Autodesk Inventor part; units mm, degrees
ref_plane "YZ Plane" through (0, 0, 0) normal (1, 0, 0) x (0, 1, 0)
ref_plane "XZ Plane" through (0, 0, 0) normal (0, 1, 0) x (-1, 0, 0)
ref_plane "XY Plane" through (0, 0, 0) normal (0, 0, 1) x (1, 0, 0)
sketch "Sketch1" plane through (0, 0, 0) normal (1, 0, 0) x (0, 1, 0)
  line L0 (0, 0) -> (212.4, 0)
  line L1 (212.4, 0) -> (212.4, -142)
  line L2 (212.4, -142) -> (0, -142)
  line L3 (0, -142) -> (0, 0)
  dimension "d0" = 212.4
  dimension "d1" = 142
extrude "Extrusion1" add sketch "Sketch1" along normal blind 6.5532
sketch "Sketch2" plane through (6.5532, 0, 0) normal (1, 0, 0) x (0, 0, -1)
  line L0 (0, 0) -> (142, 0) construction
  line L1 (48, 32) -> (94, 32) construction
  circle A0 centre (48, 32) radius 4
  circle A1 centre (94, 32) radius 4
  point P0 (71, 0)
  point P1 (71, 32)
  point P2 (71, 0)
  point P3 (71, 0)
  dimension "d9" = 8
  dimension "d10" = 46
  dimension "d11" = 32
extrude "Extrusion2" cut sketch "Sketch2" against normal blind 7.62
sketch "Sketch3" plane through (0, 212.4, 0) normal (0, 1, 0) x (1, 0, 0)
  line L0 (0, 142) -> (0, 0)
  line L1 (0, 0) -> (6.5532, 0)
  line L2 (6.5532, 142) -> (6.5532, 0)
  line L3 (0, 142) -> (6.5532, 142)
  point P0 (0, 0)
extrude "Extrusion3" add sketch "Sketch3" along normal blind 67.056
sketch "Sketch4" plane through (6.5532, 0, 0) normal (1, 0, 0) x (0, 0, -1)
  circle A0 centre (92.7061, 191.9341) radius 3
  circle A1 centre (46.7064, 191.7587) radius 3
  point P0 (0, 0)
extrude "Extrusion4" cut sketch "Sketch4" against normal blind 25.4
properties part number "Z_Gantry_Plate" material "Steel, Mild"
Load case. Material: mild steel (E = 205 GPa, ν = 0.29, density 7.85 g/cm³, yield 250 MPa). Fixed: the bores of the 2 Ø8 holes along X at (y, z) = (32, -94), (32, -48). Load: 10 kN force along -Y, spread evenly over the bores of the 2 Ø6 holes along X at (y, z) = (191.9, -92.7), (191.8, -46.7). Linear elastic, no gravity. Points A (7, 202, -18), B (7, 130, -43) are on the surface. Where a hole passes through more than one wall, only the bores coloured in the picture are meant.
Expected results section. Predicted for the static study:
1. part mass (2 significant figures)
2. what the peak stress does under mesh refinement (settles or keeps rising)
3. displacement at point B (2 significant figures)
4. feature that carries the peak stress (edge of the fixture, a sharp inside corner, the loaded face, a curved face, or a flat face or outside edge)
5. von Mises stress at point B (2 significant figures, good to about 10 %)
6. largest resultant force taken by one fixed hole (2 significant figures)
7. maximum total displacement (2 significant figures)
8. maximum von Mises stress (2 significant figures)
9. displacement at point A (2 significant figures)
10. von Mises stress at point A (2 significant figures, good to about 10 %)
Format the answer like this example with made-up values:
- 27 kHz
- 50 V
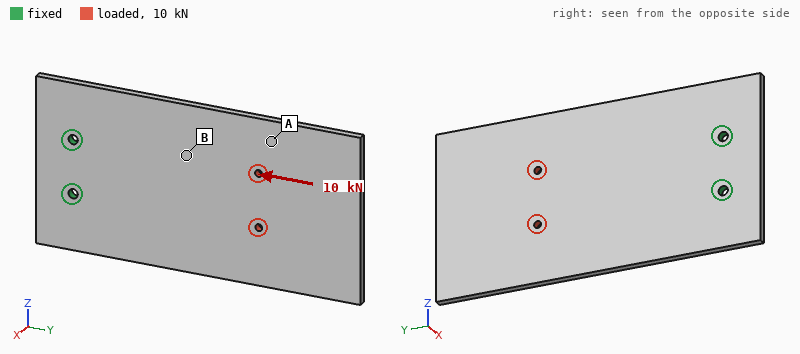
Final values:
- 2.0 kg
- settles
- 7.6 µm
- the loaded face
- 13 MPa
- 5.3 kN
- 13 µm
- 72 MPa
- 10 µm
- 5.2 MPa
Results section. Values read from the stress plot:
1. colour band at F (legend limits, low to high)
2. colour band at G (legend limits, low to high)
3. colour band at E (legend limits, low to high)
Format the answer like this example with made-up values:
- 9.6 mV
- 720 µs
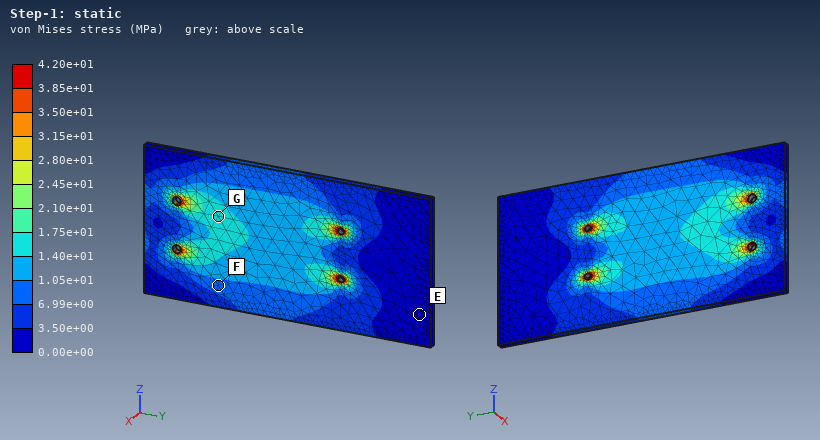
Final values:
- 6.99e+00 to 1.05e+01 MPa
- 1.40e+01 to 1.75e+01 MPa
- 0.00e+00 to 3.50e+00 MPa
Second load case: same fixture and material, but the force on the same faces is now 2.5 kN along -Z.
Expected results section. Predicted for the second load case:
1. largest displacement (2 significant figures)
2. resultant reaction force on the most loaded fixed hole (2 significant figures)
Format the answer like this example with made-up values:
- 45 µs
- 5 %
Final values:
- 70 µm
- 7.9 kN
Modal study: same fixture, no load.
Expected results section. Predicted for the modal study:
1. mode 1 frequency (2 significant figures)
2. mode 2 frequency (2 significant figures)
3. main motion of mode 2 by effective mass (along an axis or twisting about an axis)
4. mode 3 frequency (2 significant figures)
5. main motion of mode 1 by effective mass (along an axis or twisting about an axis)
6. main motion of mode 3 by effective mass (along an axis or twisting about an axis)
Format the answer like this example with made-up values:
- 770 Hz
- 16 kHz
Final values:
- 86 Hz
- 320 Hz
- twisting about Y
- 530 Hz
- along X
- along X
